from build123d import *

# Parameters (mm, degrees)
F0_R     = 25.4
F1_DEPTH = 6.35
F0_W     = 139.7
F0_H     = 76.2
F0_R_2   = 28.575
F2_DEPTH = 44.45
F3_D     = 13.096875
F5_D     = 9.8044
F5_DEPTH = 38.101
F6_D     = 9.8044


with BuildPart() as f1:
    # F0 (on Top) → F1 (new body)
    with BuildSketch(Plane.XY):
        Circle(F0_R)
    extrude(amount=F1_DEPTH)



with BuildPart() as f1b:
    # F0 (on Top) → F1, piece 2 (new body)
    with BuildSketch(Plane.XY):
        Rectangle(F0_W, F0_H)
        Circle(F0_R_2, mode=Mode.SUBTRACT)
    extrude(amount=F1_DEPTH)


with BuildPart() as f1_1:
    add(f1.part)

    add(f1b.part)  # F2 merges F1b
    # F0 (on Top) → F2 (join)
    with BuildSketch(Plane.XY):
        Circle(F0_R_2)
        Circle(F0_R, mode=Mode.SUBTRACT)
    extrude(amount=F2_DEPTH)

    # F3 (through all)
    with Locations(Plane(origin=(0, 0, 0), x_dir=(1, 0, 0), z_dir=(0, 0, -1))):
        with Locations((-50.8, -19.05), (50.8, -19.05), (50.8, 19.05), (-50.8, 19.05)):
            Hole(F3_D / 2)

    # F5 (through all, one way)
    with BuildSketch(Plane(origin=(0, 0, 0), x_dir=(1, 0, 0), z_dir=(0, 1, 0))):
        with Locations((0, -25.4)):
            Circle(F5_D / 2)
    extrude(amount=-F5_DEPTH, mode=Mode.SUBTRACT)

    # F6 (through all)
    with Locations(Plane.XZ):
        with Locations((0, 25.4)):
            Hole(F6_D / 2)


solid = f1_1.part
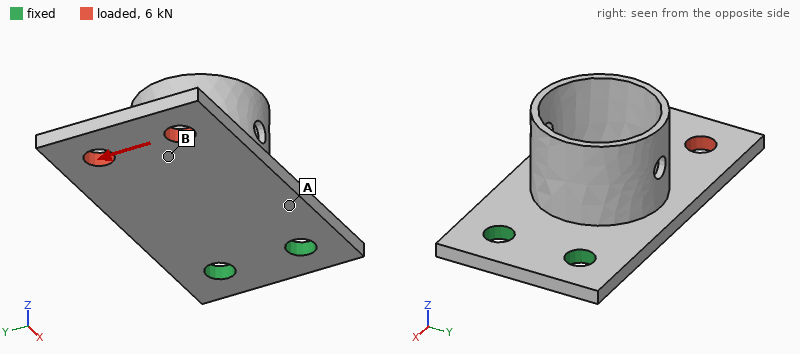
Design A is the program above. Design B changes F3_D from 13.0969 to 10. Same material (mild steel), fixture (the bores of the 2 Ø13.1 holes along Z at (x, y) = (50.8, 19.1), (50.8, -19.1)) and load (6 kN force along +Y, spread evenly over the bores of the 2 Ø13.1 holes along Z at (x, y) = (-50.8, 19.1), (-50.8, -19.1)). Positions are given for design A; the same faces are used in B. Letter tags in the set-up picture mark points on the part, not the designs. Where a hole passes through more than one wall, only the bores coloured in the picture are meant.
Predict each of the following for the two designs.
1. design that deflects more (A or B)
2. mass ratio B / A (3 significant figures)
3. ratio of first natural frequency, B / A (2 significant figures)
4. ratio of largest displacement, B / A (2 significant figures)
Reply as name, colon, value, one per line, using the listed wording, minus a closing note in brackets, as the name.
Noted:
design that deflects more: B
mass ratio B / A: 1.02
ratio of first natural frequency, B / A: 0.94
ratio of largest displacement, B / A: 1.1
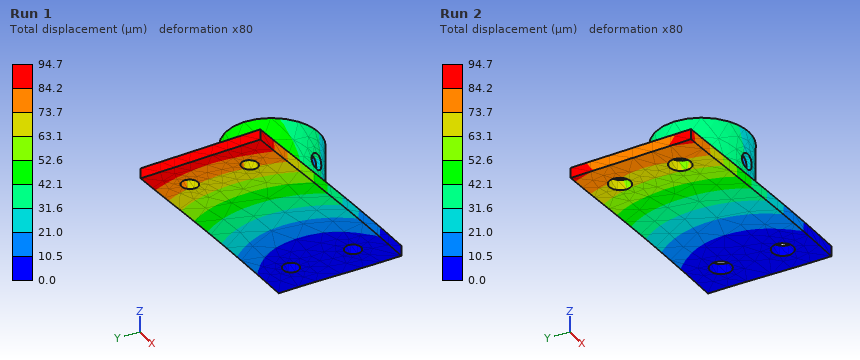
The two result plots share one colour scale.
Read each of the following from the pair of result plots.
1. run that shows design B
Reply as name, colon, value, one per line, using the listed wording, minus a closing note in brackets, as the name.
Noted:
run that shows design B: Run 1
